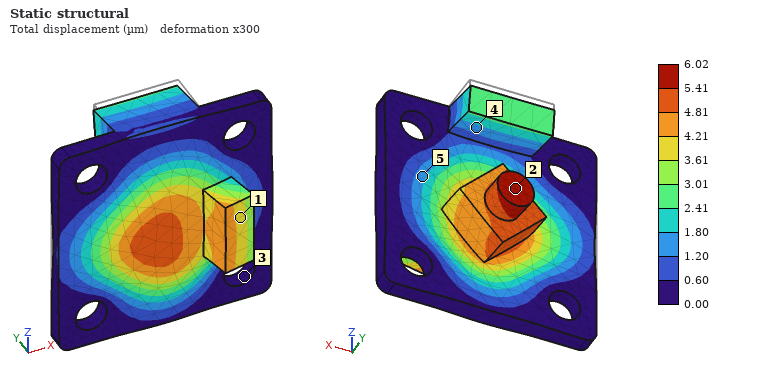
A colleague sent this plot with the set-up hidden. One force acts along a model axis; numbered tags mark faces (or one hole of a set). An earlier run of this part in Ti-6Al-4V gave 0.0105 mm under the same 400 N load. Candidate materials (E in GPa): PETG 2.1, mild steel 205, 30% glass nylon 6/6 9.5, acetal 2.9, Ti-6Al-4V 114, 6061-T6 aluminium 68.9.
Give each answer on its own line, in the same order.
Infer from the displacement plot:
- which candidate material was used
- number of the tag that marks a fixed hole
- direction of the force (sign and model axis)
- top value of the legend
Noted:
mild steel
3
-Y
6.02 µm
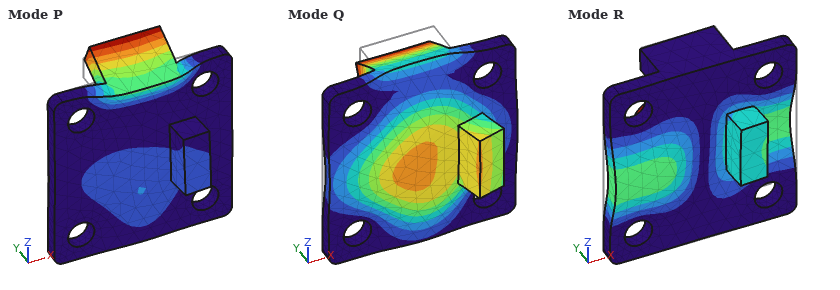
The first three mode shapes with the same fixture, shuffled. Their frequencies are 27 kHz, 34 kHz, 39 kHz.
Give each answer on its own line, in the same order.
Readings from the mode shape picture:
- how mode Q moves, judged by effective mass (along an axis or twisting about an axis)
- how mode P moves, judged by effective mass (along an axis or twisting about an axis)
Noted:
along Y
along Y
